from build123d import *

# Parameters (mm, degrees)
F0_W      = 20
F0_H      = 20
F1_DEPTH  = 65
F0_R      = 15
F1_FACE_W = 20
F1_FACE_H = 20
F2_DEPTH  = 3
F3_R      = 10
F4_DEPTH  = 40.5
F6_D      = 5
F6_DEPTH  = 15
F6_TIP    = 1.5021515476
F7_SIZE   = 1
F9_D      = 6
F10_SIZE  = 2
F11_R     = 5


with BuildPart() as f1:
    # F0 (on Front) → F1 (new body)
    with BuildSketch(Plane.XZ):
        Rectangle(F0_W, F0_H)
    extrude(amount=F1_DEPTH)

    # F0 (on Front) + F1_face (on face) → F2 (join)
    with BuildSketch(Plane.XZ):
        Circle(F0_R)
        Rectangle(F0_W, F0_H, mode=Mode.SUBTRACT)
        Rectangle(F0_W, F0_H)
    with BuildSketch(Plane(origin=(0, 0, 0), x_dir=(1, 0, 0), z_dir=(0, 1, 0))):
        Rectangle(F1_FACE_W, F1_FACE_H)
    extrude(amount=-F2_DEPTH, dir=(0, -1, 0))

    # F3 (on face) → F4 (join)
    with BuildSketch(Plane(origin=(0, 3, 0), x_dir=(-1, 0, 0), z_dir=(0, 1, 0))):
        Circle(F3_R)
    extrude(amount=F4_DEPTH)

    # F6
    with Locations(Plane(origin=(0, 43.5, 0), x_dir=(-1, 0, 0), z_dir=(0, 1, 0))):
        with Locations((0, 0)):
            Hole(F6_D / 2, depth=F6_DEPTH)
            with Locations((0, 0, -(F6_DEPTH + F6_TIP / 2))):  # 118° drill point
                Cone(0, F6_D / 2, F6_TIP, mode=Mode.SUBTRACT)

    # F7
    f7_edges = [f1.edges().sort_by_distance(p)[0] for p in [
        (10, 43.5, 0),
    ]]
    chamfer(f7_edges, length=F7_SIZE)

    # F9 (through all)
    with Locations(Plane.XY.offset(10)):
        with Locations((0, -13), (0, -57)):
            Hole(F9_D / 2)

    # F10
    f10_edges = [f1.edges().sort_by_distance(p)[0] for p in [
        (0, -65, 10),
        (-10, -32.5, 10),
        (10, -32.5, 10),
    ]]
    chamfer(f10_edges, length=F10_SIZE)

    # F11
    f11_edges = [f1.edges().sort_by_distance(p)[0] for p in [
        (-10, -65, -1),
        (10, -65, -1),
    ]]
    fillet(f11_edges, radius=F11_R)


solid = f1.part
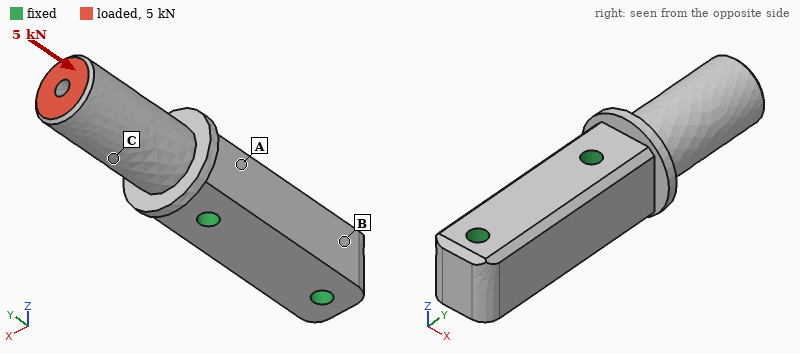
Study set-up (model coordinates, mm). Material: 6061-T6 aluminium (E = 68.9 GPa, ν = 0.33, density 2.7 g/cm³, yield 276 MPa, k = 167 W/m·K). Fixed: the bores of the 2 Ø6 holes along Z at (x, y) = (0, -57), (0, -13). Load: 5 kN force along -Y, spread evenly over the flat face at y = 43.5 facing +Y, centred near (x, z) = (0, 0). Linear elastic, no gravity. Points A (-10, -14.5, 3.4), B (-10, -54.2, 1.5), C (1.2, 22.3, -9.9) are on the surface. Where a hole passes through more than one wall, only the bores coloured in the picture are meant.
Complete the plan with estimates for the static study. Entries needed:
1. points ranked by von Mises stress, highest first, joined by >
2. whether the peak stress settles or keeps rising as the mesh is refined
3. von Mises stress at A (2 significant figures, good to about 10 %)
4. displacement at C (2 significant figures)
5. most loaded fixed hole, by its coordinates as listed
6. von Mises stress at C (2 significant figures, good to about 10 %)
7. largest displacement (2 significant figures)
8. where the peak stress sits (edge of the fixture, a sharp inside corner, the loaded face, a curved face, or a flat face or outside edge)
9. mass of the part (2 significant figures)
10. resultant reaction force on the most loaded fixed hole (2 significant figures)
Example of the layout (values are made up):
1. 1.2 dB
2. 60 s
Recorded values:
1. C > A > B
2. keeps rising
3. 6.4 MPa
4. 7.7 µm
5. (0, -13)
6. 16 MPa
7. 13 µm
8. edge of the fixture
9. 100 g
10. 4.7 kN
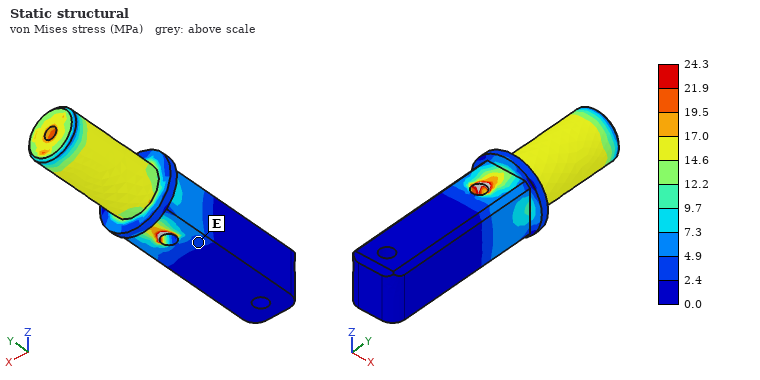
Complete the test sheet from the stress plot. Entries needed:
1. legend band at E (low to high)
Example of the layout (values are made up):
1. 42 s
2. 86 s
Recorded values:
1. 2.4 to 4.9 MPa
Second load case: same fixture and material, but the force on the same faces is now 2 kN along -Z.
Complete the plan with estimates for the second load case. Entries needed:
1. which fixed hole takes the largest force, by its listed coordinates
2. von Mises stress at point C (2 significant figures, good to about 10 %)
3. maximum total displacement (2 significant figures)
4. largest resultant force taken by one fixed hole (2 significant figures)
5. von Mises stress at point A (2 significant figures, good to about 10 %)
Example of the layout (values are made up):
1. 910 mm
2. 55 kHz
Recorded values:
1. (0, -13)
2. 54 MPa
3. 0.19 mm
4. 2.3 kN
5. 20 MPa
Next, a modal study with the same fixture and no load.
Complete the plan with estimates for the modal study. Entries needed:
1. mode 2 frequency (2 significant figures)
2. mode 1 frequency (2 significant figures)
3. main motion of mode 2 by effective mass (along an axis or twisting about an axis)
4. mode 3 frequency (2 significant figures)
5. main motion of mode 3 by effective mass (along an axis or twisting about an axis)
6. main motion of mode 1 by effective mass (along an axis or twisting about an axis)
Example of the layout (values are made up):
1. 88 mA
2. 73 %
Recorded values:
1. 4900 Hz
2. 4300 Hz
3. along Z
4. 15 kHz
5. twisting about Y
6. along X
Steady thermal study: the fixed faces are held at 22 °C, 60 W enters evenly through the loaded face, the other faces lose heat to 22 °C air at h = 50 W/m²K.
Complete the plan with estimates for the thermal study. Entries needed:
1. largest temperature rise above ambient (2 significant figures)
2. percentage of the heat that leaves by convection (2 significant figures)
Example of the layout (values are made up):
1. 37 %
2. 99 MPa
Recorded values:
1. 59 K
2. 9.9 %
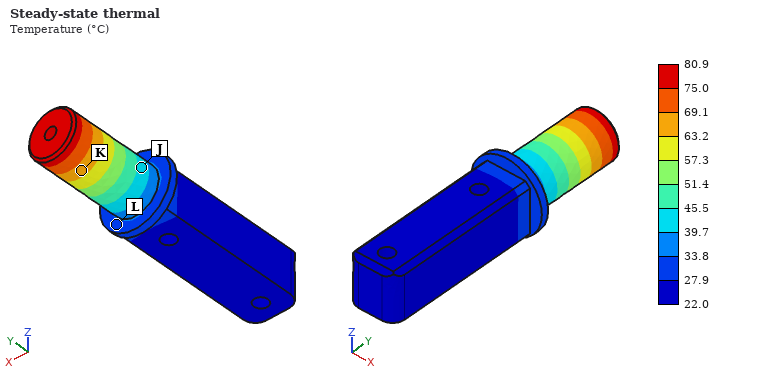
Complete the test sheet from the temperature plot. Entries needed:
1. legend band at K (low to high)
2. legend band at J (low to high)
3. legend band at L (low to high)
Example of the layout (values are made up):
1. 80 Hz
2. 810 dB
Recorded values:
1. 63.2 to 69.1 °C
2. 39.7 to 45.5 °C
3. 27.9 to 33.8 °C
